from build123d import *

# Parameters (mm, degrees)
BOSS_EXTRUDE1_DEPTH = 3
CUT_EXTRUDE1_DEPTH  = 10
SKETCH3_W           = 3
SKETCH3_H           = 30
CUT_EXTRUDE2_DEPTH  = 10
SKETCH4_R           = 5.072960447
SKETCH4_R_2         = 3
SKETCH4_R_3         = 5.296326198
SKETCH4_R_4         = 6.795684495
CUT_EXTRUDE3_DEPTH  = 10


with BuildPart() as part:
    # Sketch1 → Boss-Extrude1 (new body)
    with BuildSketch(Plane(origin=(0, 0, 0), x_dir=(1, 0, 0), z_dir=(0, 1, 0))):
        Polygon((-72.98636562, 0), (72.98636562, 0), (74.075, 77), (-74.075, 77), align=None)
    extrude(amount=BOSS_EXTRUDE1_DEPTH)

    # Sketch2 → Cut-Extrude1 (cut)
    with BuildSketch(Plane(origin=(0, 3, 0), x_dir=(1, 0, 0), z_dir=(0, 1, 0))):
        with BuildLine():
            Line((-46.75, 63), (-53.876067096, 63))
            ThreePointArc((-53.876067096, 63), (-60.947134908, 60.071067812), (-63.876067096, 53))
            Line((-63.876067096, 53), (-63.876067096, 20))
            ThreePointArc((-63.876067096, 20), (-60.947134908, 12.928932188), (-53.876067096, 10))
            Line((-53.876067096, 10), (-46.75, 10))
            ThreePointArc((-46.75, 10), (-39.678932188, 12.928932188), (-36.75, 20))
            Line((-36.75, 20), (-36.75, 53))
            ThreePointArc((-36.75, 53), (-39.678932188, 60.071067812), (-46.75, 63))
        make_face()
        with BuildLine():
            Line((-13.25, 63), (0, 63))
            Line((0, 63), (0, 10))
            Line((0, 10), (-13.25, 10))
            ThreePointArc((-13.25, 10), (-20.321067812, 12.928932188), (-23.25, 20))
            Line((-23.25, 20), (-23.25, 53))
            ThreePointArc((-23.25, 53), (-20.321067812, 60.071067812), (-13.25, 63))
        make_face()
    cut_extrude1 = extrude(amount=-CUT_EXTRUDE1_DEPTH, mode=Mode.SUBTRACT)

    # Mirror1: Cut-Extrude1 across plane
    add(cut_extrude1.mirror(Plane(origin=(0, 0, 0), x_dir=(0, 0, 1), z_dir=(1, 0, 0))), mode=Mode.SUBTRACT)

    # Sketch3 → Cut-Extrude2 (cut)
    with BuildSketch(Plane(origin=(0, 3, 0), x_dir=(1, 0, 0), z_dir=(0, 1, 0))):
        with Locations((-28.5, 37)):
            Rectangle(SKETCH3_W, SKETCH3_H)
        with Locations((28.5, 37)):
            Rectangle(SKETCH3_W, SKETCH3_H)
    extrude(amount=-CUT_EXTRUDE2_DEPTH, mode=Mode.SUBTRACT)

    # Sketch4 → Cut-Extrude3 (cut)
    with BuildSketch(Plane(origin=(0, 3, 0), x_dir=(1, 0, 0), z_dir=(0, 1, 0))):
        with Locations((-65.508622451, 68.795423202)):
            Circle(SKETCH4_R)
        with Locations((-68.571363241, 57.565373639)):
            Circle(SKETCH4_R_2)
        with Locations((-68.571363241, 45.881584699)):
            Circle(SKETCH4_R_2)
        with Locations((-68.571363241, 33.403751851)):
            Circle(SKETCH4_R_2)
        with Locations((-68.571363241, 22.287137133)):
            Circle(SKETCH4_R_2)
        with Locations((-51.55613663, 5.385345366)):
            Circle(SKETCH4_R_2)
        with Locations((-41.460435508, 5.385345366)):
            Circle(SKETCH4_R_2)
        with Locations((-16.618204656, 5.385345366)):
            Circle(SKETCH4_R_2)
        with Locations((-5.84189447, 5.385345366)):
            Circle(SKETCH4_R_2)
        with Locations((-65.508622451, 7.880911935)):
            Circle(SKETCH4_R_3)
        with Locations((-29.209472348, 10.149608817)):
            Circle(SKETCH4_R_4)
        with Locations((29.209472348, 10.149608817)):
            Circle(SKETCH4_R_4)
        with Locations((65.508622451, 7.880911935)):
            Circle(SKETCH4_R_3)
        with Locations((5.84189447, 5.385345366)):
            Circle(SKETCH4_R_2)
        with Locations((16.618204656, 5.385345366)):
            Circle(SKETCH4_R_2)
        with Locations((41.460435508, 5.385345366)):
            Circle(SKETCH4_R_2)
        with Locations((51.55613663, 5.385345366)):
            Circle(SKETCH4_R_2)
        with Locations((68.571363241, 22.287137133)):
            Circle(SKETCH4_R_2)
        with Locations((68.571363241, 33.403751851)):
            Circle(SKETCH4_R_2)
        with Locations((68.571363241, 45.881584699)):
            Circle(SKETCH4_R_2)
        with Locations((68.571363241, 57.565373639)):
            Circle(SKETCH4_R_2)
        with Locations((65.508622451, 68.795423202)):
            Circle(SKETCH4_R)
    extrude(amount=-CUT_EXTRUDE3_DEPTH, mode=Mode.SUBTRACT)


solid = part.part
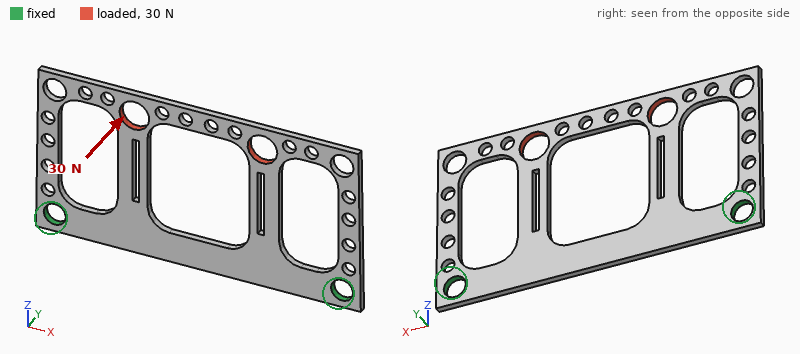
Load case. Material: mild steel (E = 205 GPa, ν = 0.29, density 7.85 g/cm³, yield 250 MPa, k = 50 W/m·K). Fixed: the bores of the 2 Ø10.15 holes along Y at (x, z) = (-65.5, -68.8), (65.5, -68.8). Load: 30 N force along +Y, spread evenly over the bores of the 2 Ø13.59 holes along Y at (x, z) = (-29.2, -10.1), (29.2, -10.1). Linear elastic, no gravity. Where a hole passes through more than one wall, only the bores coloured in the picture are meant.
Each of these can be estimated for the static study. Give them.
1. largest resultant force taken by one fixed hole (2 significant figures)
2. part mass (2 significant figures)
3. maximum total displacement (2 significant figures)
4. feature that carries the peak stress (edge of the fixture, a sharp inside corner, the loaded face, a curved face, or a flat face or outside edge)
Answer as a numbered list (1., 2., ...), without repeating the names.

1. 15 N
2. 120 g
3. 0.23 mm
4. a curved face
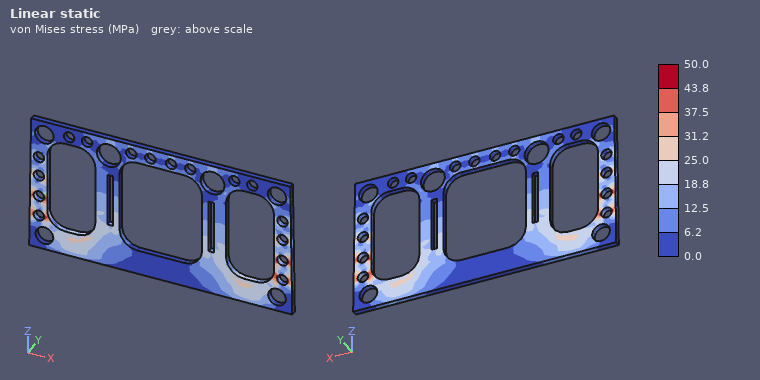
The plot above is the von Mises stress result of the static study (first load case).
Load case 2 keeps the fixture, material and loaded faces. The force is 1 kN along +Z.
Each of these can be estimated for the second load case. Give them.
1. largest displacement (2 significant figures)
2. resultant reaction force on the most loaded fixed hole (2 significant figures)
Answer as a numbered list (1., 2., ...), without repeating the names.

1. 25 µm
2. 510 N
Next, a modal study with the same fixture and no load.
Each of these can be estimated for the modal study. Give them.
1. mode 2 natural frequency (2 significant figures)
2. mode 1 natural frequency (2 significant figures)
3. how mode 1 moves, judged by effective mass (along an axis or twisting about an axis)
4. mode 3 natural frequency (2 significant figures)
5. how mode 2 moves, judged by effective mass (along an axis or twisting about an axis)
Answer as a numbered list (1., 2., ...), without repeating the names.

1. 600 Hz
2. 340 Hz
3. along Y
4. 900 Hz
5. twisting about Z
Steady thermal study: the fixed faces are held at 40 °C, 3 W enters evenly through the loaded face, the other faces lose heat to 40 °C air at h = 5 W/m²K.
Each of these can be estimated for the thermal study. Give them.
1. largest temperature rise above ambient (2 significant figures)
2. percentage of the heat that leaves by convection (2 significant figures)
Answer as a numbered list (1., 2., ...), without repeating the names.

1. 37 K
2. 37 %
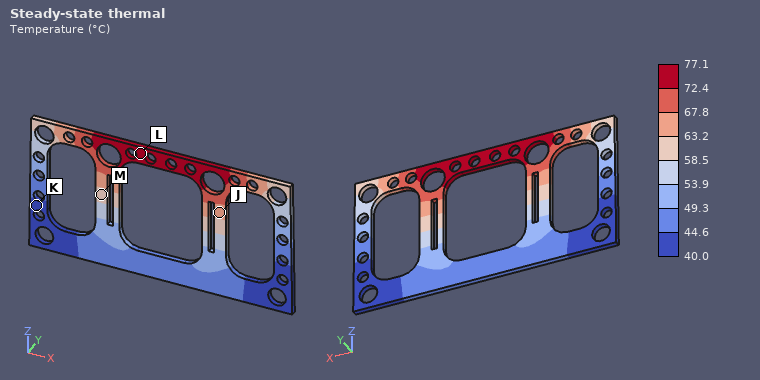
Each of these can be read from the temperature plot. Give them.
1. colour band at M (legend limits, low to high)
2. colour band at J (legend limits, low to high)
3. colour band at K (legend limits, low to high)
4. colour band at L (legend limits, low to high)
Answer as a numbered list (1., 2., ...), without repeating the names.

1. 58.5 to 63.2 °C
2. 63.2 to 67.8 °C
3. 40.0 to 44.6 °C
4. 72.4 to 77.1 °C
